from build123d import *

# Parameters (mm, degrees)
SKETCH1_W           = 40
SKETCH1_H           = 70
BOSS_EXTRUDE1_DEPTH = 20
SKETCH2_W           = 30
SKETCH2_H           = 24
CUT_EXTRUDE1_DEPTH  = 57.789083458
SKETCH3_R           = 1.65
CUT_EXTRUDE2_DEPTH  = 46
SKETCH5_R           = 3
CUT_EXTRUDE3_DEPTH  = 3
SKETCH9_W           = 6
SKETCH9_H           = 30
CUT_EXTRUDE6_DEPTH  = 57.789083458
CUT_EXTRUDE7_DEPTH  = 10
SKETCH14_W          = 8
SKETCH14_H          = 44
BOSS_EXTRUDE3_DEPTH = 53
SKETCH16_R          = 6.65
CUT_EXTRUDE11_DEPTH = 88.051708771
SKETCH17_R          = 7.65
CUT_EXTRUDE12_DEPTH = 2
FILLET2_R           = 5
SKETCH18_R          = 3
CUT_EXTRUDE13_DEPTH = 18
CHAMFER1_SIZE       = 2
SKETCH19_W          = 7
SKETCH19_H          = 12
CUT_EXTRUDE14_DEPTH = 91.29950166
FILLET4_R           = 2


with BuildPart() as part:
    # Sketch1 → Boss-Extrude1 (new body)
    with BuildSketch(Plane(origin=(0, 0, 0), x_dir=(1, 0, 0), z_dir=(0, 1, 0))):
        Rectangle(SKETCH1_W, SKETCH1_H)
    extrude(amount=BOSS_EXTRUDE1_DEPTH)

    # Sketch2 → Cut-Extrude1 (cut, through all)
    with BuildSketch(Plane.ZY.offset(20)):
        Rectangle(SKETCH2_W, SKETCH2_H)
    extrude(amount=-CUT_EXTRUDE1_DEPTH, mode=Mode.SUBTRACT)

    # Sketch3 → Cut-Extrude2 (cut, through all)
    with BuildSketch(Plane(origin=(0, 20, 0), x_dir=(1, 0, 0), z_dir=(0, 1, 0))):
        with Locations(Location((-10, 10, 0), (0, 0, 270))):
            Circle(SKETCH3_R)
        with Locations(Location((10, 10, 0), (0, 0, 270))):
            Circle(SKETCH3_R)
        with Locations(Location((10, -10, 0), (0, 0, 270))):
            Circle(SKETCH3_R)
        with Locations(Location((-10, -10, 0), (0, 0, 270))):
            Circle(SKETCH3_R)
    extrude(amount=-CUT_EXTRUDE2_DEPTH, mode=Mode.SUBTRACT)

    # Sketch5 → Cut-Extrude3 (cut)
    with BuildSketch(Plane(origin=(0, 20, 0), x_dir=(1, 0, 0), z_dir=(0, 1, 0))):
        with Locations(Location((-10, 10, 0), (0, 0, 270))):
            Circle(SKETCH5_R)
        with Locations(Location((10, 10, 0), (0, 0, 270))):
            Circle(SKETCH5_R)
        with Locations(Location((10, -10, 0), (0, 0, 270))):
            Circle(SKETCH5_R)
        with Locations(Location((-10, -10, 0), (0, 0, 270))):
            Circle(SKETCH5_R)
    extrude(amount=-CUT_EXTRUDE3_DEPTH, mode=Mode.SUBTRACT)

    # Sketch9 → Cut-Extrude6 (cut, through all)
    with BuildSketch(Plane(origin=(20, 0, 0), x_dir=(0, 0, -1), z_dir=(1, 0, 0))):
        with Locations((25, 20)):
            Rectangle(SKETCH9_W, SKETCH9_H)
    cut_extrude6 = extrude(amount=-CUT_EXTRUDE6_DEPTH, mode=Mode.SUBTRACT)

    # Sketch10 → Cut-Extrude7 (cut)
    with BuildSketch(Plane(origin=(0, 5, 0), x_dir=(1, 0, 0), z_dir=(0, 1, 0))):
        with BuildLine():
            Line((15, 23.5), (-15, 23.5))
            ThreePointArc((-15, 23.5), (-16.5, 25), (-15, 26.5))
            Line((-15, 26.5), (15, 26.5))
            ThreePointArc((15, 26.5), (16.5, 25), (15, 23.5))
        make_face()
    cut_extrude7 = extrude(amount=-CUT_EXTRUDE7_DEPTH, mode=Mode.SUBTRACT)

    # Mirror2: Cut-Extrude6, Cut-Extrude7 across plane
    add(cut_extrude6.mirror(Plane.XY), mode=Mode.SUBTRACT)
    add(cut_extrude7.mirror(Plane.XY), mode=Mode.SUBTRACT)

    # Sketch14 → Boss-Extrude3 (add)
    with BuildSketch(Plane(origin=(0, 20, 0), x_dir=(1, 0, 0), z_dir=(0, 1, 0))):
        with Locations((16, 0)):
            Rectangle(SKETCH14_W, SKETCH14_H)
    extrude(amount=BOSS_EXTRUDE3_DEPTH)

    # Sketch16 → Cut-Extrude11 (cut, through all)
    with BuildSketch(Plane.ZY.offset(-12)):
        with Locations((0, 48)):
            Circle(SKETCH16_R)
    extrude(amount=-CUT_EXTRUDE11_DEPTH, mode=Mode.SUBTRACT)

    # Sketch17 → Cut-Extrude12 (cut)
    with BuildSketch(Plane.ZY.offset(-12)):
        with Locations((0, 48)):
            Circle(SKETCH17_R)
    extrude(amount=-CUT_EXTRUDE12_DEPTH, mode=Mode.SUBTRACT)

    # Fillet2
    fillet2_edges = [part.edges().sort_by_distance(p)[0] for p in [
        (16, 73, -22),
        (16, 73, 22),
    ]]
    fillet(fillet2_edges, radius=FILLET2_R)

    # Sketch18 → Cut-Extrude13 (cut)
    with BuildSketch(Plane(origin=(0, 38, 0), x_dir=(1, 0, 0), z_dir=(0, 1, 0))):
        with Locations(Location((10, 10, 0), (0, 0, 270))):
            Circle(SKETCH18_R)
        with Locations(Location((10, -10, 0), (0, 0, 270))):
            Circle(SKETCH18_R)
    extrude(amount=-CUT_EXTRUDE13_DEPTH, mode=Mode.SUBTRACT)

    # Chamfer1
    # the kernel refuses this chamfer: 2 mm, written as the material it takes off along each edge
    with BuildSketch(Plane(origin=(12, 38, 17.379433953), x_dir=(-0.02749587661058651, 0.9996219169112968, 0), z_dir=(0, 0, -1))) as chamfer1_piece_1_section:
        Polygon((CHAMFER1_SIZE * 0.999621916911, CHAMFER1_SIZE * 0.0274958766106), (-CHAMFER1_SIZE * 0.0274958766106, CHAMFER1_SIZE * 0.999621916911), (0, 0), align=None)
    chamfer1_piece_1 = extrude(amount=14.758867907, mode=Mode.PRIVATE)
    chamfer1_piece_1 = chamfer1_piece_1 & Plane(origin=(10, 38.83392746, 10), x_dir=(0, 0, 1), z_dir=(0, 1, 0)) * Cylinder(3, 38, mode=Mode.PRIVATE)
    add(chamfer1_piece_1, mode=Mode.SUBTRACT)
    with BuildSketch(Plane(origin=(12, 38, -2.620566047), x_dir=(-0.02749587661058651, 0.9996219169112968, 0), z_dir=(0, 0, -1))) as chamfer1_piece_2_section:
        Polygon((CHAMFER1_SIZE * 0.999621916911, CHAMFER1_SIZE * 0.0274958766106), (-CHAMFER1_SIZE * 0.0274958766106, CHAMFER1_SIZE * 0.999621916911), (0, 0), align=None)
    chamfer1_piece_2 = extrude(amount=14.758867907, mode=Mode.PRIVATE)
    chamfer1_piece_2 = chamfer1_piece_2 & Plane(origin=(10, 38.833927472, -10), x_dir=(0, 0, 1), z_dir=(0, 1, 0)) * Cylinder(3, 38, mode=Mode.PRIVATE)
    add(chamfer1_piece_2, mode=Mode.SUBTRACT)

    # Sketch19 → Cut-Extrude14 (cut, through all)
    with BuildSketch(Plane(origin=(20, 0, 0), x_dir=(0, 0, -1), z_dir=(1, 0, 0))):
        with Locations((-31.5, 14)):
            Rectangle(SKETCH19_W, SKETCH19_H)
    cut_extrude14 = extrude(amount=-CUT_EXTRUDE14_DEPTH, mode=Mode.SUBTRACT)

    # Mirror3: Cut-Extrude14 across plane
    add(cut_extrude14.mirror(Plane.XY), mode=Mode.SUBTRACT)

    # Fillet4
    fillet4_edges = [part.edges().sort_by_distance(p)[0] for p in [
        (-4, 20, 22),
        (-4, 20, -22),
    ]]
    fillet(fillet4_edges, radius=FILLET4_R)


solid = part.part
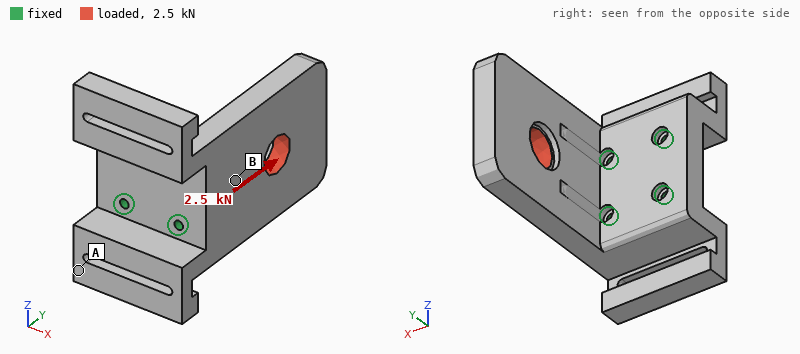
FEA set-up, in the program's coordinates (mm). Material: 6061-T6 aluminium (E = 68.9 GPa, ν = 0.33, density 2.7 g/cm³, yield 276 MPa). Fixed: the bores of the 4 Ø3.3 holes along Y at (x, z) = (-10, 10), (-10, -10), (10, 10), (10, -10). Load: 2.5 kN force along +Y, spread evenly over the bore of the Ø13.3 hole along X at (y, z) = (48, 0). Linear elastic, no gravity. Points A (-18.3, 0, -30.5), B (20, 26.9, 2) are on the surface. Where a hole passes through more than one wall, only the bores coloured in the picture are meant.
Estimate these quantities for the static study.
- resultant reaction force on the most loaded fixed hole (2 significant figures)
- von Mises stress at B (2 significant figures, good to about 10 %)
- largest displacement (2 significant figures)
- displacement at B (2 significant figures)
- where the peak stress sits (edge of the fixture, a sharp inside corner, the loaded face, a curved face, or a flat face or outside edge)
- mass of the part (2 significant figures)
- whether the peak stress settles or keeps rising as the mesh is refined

1.5 kN
12 MPa
70 µm
16 µm
edge of the fixture
120 g
keeps rising
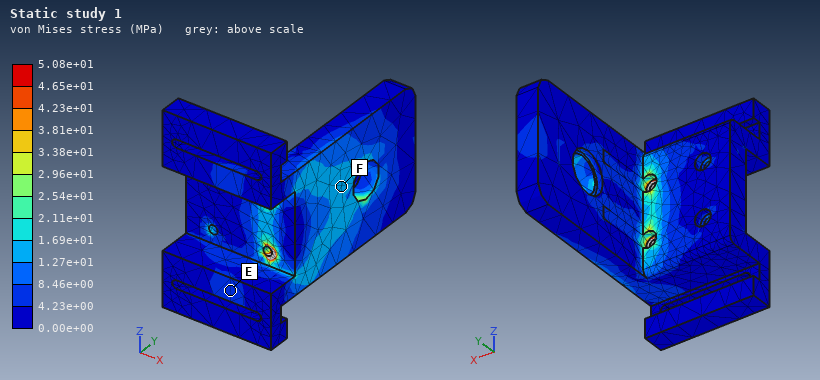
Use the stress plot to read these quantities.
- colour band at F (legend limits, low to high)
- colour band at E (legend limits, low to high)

1.27e+01 to 1.69e+01 MPa
4.23e+00 to 8.46e+00 MPa
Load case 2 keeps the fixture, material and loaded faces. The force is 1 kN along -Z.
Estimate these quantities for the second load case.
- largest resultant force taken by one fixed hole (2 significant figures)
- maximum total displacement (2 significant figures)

1.5 kN
40 µm
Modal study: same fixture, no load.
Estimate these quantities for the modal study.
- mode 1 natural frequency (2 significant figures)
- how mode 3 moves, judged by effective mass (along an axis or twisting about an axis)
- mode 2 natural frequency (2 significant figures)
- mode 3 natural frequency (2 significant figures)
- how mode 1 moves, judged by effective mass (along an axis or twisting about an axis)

1700 Hz
along Y
3900 Hz
4700 Hz
along X
